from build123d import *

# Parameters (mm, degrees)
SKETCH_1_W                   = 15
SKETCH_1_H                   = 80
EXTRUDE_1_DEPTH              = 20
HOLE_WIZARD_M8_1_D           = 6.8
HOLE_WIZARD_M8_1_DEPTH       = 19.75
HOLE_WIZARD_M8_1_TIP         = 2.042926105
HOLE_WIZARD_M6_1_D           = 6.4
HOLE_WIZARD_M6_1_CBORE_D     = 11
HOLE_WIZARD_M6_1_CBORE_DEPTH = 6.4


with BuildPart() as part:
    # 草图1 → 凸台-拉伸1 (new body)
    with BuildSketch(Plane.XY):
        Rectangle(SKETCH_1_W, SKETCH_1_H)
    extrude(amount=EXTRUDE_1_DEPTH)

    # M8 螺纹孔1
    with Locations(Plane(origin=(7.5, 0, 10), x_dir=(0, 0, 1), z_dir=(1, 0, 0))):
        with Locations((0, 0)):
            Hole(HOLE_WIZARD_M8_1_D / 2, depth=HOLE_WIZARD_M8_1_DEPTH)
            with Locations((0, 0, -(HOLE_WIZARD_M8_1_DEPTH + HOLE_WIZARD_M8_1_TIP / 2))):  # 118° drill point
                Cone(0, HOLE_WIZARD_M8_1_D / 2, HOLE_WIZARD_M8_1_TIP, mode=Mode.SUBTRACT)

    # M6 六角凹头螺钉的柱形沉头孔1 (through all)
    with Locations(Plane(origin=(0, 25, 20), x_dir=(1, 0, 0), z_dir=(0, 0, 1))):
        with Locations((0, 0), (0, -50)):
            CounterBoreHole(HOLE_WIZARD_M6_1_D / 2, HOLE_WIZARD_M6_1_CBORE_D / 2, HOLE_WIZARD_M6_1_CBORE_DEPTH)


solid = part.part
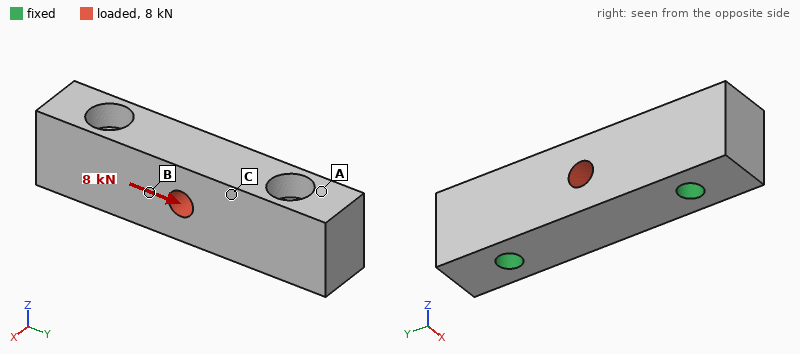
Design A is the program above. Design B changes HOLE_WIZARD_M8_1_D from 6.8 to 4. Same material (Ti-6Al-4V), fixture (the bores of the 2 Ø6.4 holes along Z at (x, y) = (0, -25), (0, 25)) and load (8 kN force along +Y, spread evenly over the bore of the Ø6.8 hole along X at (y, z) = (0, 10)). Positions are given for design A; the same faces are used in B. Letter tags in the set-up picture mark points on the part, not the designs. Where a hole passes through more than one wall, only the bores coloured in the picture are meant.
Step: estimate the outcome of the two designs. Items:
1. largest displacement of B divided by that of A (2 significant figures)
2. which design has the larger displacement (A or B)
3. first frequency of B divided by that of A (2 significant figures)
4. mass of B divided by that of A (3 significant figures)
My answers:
1.1
B
1.00
1.02
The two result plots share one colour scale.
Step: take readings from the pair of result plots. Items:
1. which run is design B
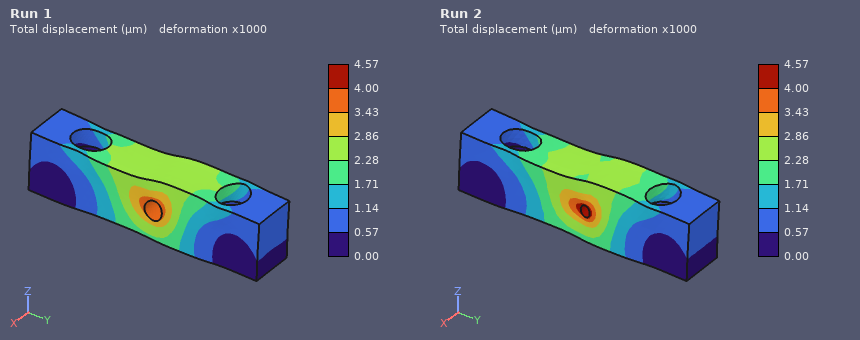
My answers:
Run 2
